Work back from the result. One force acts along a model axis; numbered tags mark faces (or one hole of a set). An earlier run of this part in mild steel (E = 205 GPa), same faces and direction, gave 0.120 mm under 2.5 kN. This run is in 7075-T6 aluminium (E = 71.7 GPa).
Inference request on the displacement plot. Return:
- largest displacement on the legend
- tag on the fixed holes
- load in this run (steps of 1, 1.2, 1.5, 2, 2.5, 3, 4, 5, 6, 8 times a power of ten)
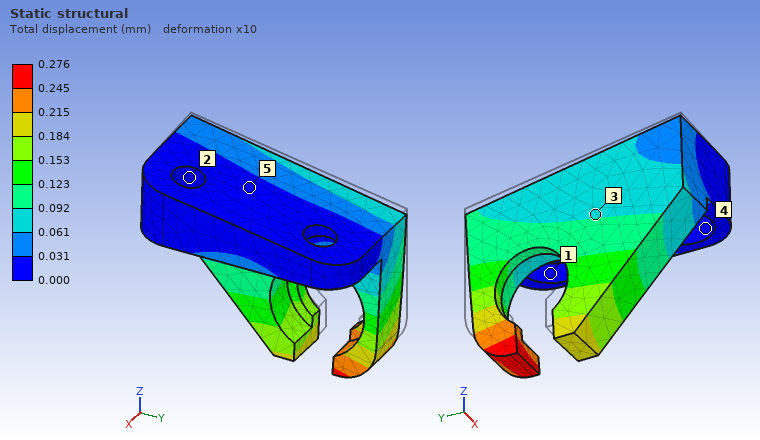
0.276 mm
2
2 kN
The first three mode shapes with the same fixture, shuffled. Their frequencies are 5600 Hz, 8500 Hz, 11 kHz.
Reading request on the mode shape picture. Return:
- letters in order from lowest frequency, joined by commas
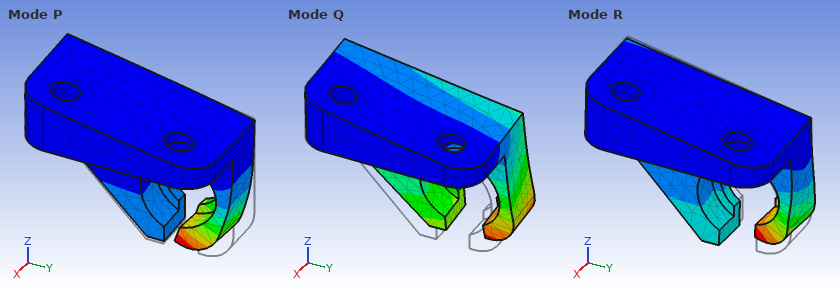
Q, P, R
